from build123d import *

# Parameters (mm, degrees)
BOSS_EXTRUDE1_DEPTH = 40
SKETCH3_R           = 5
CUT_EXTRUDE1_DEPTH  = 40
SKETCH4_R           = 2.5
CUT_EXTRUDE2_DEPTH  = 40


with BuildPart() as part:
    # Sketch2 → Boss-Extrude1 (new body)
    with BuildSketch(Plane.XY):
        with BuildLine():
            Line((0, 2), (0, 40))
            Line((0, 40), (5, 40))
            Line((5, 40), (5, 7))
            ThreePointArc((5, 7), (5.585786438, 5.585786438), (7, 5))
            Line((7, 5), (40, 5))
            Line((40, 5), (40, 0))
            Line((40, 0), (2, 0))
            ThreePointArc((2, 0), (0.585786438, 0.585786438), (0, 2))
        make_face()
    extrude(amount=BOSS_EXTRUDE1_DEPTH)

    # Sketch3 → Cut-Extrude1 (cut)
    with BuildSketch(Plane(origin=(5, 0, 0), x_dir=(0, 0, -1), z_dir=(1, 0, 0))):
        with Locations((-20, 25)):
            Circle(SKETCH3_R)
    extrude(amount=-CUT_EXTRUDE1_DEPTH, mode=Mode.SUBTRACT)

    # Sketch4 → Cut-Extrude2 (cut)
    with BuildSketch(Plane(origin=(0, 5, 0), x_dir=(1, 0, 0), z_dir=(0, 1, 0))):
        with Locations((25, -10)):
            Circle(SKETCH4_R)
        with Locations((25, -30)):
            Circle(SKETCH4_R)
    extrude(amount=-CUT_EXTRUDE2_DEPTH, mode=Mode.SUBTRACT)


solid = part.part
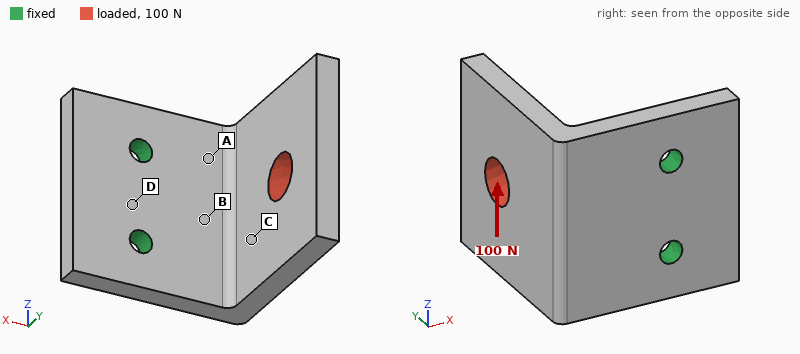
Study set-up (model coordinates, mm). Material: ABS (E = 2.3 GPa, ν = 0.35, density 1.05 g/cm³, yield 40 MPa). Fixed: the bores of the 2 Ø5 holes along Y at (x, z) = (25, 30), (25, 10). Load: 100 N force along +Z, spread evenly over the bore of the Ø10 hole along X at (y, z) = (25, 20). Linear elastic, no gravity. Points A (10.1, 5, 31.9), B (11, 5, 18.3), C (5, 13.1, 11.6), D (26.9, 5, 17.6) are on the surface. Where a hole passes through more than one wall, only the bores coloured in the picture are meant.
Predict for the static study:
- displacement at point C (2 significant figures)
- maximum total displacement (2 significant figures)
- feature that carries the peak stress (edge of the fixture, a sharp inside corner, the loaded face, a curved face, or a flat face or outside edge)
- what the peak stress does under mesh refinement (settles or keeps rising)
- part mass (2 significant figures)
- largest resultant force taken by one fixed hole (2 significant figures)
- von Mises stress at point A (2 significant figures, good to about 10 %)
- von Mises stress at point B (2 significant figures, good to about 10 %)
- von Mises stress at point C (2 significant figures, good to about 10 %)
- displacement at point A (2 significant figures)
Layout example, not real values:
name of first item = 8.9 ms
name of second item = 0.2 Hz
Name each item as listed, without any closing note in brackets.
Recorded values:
displacement at point C = 0.25 mm
maximum total displacement = 0.75 mm
feature that carries the peak stress = edge of the fixture
what the peak stress does under mesh refinement = keeps rising
part mass = 15 g
largest resultant force taken by one fixed hole = 140 N
von Mises stress at point A = 6.9 MPa
von Mises stress at point B = 7.9 MPa
von Mises stress at point C = 3.2 MPa
displacement at point A = 0.13 mm
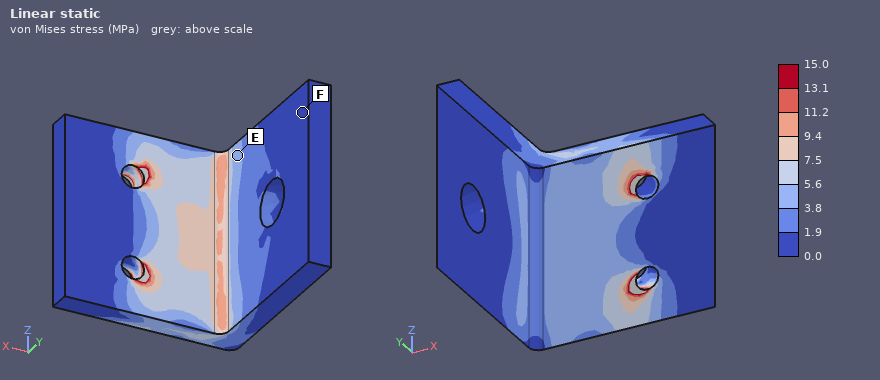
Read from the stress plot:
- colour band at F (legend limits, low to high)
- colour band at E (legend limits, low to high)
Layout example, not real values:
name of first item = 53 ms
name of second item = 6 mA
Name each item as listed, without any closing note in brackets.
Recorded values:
colour band at F = 0.0 to 1.9 MPa
colour band at E = 3.8 to 5.6 MPa
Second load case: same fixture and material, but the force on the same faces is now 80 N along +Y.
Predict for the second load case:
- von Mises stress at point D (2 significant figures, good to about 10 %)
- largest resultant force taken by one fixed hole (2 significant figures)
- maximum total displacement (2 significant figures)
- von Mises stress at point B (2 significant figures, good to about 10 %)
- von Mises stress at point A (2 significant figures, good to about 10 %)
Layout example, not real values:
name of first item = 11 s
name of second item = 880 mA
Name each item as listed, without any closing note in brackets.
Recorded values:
von Mises stress at point D = 2.4 MPa
largest resultant force taken by one fixed hole = 40 N
maximum total displacement = 0.80 mm
von Mises stress at point B = 3.7 MPa
von Mises stress at point A = 3.2 MPa
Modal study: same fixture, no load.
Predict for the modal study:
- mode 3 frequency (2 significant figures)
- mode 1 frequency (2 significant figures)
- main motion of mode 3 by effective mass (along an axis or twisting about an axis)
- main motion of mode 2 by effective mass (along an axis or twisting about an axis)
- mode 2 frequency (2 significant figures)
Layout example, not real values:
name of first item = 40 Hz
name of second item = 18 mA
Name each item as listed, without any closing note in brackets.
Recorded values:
mode 3 frequency = 1400 Hz
mode 1 frequency = 470 Hz
main motion of mode 3 by effective mass = along Y
main motion of mode 2 by effective mass = along Z
mode 2 frequency = 830 Hz
